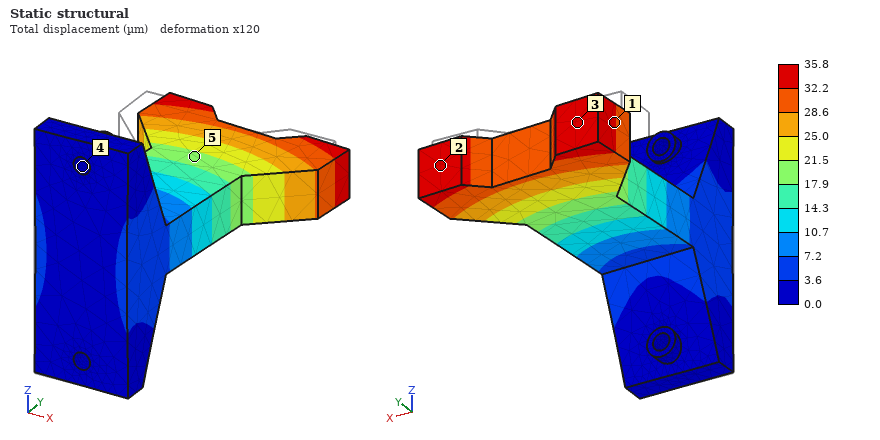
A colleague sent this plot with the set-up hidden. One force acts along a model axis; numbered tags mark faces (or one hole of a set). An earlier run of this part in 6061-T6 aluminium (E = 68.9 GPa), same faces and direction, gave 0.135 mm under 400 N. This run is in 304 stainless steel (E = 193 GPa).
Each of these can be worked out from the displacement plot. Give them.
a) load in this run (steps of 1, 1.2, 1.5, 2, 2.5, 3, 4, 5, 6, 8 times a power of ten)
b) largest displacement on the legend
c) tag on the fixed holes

300 N
35.8 µm
4
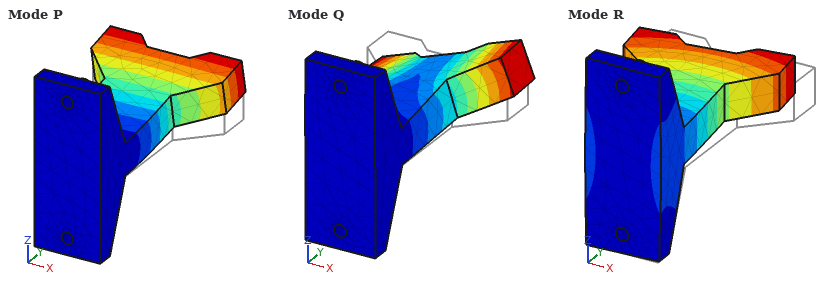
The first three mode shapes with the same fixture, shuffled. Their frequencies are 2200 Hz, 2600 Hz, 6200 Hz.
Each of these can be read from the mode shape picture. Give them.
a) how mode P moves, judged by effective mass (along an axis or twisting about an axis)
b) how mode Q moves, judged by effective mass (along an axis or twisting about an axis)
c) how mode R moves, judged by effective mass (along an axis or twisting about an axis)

along Z
twisting about Y
along X
